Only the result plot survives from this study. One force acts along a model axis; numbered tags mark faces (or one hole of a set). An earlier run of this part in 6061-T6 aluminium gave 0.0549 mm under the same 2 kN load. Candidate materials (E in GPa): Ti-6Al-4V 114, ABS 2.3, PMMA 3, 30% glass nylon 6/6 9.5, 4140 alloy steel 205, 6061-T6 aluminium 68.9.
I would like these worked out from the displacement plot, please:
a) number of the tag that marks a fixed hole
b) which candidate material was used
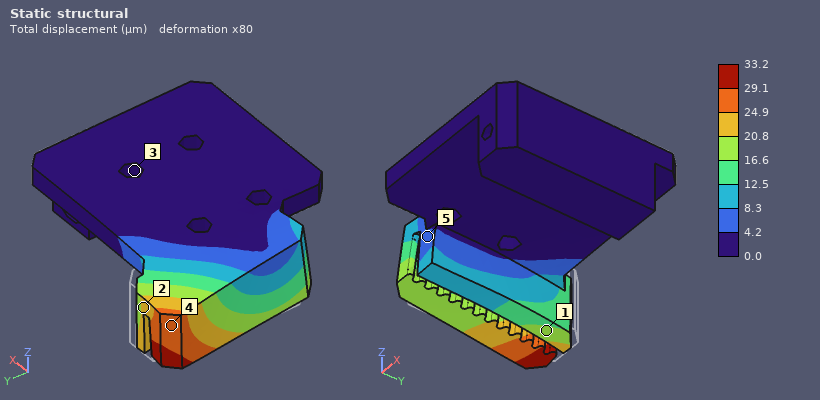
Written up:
3
Ti-6Al-4V
